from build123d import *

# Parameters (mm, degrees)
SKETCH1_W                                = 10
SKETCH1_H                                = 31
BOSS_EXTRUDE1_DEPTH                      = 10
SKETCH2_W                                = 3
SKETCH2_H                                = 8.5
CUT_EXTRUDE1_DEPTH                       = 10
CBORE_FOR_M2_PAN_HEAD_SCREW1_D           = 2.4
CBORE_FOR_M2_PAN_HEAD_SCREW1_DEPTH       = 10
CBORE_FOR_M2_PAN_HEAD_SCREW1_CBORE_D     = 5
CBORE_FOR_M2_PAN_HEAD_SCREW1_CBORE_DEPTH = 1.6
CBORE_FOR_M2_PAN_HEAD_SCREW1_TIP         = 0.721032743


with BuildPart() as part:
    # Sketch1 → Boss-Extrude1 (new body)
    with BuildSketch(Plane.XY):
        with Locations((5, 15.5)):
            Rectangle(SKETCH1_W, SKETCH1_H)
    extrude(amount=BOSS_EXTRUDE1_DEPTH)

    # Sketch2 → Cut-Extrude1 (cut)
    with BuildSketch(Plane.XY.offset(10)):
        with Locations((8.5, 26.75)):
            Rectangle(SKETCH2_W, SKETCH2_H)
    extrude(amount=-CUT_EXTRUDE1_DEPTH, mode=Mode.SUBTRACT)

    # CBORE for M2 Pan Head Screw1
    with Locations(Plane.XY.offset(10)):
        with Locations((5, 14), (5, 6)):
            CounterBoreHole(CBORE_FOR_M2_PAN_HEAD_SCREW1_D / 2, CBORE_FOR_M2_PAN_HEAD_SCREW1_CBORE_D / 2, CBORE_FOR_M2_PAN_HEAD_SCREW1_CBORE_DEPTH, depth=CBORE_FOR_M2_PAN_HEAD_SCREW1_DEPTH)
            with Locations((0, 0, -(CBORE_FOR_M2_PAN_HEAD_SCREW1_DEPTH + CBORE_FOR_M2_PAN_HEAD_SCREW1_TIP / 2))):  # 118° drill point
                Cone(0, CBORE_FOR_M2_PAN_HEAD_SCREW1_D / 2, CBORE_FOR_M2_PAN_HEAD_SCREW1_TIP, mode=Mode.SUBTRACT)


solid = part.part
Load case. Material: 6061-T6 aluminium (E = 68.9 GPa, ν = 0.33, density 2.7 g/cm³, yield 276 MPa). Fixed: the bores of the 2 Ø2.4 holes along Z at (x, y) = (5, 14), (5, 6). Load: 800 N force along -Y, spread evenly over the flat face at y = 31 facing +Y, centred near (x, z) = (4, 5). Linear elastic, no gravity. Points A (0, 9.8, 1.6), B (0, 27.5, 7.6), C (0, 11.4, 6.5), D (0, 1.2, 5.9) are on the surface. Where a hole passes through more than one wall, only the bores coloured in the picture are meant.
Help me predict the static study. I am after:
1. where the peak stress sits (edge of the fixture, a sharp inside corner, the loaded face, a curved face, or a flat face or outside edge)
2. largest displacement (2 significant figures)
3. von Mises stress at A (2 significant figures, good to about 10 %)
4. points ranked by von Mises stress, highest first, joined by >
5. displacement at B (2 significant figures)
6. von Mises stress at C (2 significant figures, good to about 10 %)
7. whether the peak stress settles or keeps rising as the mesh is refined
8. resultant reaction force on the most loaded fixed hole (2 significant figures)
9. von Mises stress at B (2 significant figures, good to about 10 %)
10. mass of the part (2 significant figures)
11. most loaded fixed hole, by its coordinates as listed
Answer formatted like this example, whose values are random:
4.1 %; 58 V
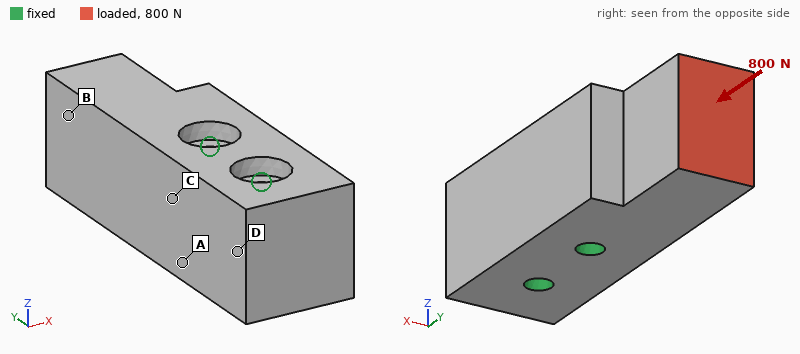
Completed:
edge of the fixture; 5.6 µm; 4.8 MPa; B > C > A > D; 4.5 µm; 8.1 MPa; keeps rising; 660 N; 11 MPa; 7.3 g; (5, 14)
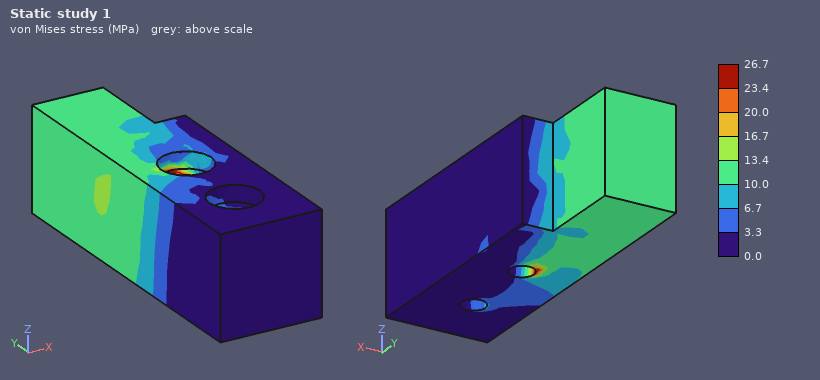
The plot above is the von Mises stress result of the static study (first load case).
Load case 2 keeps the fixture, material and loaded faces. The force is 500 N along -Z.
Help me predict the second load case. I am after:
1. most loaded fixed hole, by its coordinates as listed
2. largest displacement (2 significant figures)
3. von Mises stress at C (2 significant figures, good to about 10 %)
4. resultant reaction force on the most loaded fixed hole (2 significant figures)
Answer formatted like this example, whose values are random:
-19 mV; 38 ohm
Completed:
(5, 14); 29 µm; 13 MPa; 730 N
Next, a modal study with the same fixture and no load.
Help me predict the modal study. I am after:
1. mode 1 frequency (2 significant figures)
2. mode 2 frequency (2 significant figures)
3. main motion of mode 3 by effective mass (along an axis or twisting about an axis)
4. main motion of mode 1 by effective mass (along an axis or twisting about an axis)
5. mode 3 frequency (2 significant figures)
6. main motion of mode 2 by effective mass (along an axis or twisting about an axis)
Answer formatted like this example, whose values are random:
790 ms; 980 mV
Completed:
20 kHz; 22 kHz; twisting about Y; along X; 44 kHz; along Z
